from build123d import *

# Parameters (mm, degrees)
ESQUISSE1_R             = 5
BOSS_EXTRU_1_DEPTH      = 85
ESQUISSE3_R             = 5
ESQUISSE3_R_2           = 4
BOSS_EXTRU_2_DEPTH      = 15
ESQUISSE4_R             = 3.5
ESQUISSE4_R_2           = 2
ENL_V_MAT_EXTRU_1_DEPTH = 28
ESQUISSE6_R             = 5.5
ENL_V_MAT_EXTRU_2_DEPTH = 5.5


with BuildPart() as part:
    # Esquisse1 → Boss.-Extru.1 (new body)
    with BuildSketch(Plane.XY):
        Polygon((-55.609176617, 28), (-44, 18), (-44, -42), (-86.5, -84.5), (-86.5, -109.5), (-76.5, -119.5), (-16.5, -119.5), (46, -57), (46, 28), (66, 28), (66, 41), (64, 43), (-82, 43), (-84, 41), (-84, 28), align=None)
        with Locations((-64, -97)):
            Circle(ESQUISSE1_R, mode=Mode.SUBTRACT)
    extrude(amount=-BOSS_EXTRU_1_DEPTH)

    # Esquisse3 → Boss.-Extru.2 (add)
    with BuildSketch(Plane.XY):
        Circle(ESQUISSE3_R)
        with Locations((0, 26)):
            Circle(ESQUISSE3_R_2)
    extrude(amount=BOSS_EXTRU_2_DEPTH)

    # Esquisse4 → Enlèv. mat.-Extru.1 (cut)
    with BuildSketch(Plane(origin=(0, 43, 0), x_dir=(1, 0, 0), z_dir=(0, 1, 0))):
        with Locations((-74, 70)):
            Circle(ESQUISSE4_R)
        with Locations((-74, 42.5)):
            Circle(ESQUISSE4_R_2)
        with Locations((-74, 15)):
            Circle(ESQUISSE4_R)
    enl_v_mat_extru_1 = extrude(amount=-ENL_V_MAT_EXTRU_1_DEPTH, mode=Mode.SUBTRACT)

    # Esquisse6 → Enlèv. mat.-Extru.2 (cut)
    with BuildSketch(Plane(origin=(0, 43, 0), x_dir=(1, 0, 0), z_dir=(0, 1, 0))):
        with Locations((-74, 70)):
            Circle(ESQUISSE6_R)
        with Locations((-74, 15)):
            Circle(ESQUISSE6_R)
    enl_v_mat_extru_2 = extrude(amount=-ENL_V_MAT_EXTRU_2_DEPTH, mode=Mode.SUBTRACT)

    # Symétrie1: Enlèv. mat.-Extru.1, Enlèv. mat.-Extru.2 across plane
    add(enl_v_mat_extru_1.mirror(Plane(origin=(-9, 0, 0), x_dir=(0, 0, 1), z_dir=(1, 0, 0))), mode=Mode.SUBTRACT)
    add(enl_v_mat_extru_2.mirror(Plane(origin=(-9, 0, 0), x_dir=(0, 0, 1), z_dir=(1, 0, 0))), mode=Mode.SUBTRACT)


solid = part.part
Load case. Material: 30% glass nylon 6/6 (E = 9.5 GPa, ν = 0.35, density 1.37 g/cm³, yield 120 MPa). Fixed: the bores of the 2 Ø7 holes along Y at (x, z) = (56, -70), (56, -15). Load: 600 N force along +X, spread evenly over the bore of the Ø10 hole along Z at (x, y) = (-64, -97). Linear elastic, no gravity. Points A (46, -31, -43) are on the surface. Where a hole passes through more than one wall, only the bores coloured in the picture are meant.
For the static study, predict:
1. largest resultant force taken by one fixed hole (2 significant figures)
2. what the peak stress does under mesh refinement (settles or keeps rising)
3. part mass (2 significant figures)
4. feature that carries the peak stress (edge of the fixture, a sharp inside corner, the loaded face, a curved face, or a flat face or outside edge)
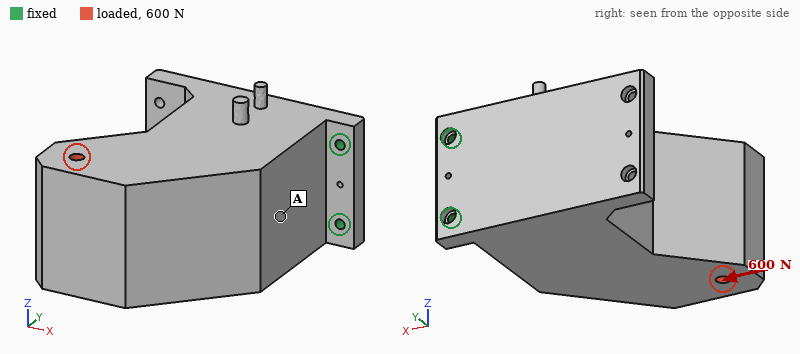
300 N
keeps rising
1.8 kg
edge of the fixture
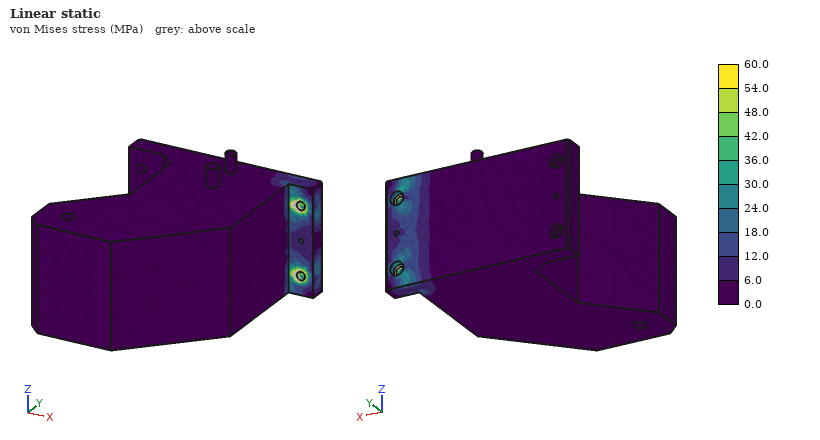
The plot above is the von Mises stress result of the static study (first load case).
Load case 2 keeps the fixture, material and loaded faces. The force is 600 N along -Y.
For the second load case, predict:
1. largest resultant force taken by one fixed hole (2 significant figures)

310 N
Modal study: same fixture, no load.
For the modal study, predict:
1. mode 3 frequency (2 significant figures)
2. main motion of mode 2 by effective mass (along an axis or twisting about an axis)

890 Hz
along Z
